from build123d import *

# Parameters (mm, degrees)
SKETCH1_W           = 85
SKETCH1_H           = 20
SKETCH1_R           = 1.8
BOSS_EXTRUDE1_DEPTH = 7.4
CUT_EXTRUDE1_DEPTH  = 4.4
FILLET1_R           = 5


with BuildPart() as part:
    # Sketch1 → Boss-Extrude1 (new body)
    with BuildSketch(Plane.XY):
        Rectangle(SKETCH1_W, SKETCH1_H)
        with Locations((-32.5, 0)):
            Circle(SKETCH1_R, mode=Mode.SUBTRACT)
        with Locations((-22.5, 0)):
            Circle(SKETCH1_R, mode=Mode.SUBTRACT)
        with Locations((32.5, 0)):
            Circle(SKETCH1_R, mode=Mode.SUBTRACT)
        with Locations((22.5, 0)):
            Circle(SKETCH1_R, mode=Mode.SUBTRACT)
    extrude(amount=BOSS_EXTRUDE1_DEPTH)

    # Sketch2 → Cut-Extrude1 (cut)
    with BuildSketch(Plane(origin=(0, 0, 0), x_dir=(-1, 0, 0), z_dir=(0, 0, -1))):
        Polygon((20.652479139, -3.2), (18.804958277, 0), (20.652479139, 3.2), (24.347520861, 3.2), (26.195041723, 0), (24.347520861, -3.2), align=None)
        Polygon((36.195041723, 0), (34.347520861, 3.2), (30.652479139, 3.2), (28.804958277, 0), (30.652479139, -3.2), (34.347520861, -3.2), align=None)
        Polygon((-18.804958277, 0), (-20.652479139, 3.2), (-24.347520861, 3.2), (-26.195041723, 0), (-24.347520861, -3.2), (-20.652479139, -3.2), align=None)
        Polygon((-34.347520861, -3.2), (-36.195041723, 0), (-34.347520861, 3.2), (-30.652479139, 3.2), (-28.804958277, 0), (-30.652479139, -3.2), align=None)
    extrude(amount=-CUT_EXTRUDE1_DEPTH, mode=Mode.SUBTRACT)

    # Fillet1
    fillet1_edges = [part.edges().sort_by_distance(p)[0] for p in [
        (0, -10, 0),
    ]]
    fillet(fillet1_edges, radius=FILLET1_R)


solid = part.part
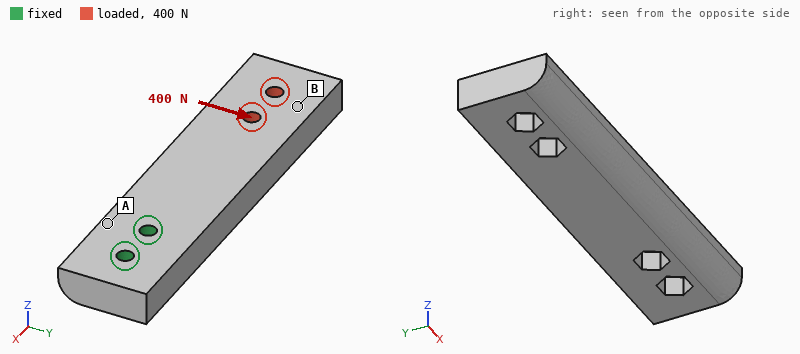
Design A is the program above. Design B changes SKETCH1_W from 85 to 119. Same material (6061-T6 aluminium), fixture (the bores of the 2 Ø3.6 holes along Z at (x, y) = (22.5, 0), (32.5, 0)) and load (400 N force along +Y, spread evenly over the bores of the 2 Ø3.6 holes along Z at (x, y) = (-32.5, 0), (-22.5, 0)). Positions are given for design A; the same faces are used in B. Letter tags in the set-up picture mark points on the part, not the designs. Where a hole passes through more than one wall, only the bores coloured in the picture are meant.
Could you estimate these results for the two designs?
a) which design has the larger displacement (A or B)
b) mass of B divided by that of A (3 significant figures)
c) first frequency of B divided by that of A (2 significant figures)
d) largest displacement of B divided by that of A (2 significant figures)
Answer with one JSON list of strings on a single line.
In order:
["B", "1.43", "0.63", "1.3"]
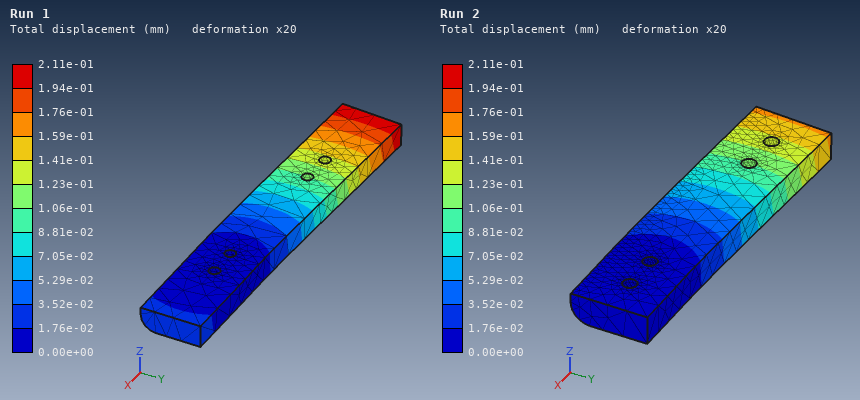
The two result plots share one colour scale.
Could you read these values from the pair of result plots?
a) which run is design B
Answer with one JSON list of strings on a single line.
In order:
["Run 1"]
